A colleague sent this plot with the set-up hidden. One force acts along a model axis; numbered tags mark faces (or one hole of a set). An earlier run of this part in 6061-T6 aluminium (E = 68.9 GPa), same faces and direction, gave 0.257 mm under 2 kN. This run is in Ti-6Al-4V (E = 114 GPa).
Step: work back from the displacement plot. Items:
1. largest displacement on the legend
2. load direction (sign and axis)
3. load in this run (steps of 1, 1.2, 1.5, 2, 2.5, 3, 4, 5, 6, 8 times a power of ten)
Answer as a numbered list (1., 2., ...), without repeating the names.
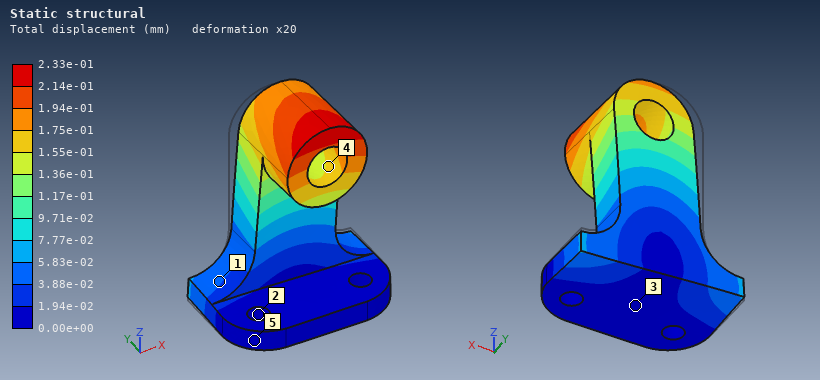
1. 2.33e-01 mm
2. +X
3. 3 kN
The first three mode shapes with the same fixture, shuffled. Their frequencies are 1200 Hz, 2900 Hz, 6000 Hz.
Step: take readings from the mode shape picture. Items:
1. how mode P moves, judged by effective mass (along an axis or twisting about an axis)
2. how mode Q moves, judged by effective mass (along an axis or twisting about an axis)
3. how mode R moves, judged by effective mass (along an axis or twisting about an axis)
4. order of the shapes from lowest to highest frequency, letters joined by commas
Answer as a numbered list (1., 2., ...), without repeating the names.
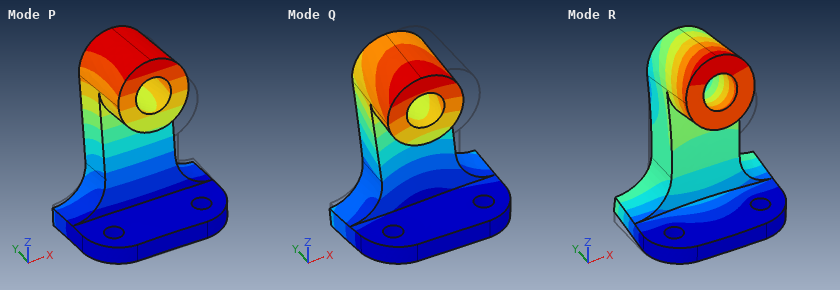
1. along Y
2. along X
3. along Z
4. P, Q, R
